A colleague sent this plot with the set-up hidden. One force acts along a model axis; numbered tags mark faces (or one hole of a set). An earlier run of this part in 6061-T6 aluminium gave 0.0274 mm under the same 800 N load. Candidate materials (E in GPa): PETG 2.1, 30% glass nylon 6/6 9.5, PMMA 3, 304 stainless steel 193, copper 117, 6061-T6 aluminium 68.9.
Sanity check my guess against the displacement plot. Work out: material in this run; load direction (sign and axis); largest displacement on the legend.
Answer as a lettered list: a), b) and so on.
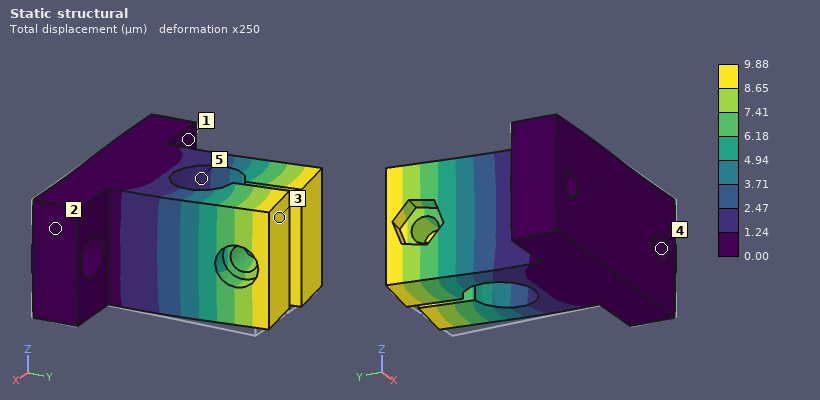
a) 304 stainless steel
b) -X
c) 9.88 µm
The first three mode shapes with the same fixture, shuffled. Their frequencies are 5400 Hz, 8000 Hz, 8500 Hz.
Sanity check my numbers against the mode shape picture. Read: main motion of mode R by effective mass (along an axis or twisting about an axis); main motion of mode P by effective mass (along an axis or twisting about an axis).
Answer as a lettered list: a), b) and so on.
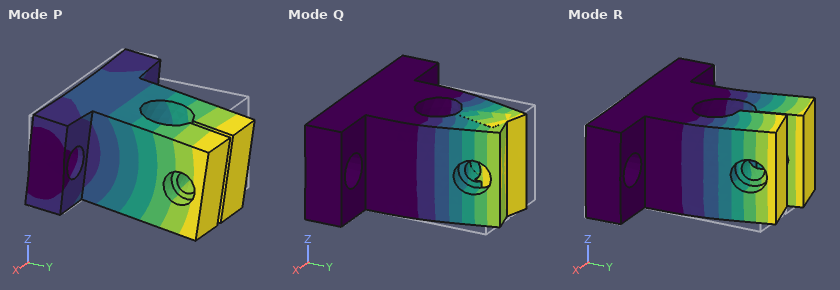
a) along X
b) along Z
